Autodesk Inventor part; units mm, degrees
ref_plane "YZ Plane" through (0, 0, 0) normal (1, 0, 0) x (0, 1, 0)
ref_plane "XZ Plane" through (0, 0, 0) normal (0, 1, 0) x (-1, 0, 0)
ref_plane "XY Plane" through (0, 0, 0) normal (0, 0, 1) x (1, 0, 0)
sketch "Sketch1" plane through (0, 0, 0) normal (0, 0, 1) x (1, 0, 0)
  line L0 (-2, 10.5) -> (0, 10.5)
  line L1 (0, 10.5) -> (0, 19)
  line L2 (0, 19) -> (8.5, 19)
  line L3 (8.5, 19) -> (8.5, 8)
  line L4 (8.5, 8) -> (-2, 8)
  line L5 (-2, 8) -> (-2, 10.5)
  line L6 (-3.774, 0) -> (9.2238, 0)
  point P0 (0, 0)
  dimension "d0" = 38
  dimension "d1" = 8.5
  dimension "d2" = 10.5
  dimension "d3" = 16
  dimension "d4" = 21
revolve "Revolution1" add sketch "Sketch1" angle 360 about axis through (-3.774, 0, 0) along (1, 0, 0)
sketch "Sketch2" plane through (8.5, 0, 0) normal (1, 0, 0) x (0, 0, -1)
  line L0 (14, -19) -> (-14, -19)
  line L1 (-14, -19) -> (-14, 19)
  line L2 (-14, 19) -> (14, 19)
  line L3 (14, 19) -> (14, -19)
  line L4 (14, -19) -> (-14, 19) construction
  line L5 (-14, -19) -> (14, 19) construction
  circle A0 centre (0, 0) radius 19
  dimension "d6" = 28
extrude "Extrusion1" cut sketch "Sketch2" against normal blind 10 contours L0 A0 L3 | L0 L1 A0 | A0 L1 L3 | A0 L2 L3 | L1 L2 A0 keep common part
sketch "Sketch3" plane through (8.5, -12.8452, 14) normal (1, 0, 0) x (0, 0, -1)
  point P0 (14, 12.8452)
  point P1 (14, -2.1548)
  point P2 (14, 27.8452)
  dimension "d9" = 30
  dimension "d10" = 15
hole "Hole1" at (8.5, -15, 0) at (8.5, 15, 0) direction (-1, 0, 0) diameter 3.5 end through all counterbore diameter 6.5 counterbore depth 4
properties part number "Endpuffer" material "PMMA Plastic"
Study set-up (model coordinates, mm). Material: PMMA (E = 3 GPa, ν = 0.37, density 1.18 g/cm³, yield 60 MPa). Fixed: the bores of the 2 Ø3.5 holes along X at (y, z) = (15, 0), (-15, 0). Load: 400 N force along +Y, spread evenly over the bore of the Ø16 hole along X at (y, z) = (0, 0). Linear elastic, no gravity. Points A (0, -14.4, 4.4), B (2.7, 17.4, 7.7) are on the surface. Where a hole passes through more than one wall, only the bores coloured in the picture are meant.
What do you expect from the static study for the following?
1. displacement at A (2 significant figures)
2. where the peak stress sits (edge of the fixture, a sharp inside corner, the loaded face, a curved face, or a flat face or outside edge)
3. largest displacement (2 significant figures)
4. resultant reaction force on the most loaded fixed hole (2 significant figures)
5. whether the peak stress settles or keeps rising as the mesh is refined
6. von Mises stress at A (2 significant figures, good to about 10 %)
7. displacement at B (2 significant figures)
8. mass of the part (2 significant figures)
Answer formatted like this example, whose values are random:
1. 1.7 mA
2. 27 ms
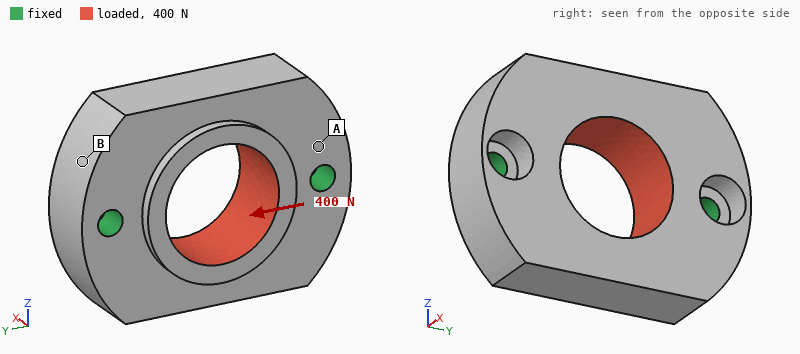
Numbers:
1. 5.6 µm
2. edge of the fixture
3. 16 µm
4. 200 N
5. keeps rising
6. 1.8 MPa
7. 10 µm
8. 7.4 g
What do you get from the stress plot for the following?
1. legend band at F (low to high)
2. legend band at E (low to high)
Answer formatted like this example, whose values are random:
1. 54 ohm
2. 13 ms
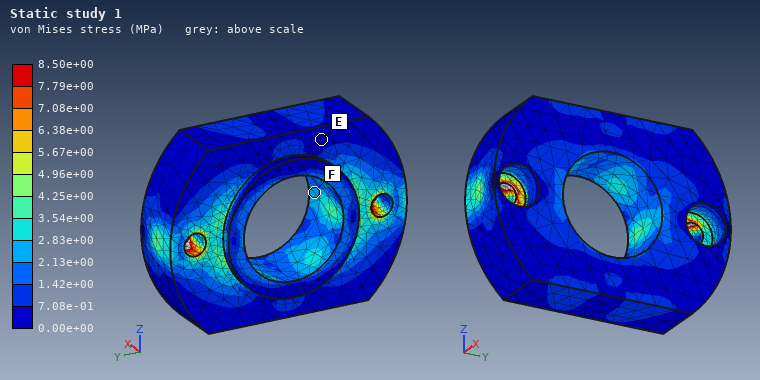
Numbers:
1. 2.13e+00 to 2.83e+00 MPa
2. 0.00e+00 to 7.08e-01 MPa
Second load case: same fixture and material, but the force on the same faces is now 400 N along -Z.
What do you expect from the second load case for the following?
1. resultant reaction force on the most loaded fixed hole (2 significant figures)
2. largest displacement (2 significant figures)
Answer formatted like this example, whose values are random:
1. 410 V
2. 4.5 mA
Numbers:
1. 200 N
2. 38 µm
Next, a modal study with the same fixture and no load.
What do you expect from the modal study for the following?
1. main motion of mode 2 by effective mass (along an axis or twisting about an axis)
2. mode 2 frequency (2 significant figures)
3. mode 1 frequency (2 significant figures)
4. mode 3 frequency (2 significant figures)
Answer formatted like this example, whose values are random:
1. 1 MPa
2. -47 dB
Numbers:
1. along X
2. 5700 Hz
3. 3500 Hz
4. 8200 Hz
